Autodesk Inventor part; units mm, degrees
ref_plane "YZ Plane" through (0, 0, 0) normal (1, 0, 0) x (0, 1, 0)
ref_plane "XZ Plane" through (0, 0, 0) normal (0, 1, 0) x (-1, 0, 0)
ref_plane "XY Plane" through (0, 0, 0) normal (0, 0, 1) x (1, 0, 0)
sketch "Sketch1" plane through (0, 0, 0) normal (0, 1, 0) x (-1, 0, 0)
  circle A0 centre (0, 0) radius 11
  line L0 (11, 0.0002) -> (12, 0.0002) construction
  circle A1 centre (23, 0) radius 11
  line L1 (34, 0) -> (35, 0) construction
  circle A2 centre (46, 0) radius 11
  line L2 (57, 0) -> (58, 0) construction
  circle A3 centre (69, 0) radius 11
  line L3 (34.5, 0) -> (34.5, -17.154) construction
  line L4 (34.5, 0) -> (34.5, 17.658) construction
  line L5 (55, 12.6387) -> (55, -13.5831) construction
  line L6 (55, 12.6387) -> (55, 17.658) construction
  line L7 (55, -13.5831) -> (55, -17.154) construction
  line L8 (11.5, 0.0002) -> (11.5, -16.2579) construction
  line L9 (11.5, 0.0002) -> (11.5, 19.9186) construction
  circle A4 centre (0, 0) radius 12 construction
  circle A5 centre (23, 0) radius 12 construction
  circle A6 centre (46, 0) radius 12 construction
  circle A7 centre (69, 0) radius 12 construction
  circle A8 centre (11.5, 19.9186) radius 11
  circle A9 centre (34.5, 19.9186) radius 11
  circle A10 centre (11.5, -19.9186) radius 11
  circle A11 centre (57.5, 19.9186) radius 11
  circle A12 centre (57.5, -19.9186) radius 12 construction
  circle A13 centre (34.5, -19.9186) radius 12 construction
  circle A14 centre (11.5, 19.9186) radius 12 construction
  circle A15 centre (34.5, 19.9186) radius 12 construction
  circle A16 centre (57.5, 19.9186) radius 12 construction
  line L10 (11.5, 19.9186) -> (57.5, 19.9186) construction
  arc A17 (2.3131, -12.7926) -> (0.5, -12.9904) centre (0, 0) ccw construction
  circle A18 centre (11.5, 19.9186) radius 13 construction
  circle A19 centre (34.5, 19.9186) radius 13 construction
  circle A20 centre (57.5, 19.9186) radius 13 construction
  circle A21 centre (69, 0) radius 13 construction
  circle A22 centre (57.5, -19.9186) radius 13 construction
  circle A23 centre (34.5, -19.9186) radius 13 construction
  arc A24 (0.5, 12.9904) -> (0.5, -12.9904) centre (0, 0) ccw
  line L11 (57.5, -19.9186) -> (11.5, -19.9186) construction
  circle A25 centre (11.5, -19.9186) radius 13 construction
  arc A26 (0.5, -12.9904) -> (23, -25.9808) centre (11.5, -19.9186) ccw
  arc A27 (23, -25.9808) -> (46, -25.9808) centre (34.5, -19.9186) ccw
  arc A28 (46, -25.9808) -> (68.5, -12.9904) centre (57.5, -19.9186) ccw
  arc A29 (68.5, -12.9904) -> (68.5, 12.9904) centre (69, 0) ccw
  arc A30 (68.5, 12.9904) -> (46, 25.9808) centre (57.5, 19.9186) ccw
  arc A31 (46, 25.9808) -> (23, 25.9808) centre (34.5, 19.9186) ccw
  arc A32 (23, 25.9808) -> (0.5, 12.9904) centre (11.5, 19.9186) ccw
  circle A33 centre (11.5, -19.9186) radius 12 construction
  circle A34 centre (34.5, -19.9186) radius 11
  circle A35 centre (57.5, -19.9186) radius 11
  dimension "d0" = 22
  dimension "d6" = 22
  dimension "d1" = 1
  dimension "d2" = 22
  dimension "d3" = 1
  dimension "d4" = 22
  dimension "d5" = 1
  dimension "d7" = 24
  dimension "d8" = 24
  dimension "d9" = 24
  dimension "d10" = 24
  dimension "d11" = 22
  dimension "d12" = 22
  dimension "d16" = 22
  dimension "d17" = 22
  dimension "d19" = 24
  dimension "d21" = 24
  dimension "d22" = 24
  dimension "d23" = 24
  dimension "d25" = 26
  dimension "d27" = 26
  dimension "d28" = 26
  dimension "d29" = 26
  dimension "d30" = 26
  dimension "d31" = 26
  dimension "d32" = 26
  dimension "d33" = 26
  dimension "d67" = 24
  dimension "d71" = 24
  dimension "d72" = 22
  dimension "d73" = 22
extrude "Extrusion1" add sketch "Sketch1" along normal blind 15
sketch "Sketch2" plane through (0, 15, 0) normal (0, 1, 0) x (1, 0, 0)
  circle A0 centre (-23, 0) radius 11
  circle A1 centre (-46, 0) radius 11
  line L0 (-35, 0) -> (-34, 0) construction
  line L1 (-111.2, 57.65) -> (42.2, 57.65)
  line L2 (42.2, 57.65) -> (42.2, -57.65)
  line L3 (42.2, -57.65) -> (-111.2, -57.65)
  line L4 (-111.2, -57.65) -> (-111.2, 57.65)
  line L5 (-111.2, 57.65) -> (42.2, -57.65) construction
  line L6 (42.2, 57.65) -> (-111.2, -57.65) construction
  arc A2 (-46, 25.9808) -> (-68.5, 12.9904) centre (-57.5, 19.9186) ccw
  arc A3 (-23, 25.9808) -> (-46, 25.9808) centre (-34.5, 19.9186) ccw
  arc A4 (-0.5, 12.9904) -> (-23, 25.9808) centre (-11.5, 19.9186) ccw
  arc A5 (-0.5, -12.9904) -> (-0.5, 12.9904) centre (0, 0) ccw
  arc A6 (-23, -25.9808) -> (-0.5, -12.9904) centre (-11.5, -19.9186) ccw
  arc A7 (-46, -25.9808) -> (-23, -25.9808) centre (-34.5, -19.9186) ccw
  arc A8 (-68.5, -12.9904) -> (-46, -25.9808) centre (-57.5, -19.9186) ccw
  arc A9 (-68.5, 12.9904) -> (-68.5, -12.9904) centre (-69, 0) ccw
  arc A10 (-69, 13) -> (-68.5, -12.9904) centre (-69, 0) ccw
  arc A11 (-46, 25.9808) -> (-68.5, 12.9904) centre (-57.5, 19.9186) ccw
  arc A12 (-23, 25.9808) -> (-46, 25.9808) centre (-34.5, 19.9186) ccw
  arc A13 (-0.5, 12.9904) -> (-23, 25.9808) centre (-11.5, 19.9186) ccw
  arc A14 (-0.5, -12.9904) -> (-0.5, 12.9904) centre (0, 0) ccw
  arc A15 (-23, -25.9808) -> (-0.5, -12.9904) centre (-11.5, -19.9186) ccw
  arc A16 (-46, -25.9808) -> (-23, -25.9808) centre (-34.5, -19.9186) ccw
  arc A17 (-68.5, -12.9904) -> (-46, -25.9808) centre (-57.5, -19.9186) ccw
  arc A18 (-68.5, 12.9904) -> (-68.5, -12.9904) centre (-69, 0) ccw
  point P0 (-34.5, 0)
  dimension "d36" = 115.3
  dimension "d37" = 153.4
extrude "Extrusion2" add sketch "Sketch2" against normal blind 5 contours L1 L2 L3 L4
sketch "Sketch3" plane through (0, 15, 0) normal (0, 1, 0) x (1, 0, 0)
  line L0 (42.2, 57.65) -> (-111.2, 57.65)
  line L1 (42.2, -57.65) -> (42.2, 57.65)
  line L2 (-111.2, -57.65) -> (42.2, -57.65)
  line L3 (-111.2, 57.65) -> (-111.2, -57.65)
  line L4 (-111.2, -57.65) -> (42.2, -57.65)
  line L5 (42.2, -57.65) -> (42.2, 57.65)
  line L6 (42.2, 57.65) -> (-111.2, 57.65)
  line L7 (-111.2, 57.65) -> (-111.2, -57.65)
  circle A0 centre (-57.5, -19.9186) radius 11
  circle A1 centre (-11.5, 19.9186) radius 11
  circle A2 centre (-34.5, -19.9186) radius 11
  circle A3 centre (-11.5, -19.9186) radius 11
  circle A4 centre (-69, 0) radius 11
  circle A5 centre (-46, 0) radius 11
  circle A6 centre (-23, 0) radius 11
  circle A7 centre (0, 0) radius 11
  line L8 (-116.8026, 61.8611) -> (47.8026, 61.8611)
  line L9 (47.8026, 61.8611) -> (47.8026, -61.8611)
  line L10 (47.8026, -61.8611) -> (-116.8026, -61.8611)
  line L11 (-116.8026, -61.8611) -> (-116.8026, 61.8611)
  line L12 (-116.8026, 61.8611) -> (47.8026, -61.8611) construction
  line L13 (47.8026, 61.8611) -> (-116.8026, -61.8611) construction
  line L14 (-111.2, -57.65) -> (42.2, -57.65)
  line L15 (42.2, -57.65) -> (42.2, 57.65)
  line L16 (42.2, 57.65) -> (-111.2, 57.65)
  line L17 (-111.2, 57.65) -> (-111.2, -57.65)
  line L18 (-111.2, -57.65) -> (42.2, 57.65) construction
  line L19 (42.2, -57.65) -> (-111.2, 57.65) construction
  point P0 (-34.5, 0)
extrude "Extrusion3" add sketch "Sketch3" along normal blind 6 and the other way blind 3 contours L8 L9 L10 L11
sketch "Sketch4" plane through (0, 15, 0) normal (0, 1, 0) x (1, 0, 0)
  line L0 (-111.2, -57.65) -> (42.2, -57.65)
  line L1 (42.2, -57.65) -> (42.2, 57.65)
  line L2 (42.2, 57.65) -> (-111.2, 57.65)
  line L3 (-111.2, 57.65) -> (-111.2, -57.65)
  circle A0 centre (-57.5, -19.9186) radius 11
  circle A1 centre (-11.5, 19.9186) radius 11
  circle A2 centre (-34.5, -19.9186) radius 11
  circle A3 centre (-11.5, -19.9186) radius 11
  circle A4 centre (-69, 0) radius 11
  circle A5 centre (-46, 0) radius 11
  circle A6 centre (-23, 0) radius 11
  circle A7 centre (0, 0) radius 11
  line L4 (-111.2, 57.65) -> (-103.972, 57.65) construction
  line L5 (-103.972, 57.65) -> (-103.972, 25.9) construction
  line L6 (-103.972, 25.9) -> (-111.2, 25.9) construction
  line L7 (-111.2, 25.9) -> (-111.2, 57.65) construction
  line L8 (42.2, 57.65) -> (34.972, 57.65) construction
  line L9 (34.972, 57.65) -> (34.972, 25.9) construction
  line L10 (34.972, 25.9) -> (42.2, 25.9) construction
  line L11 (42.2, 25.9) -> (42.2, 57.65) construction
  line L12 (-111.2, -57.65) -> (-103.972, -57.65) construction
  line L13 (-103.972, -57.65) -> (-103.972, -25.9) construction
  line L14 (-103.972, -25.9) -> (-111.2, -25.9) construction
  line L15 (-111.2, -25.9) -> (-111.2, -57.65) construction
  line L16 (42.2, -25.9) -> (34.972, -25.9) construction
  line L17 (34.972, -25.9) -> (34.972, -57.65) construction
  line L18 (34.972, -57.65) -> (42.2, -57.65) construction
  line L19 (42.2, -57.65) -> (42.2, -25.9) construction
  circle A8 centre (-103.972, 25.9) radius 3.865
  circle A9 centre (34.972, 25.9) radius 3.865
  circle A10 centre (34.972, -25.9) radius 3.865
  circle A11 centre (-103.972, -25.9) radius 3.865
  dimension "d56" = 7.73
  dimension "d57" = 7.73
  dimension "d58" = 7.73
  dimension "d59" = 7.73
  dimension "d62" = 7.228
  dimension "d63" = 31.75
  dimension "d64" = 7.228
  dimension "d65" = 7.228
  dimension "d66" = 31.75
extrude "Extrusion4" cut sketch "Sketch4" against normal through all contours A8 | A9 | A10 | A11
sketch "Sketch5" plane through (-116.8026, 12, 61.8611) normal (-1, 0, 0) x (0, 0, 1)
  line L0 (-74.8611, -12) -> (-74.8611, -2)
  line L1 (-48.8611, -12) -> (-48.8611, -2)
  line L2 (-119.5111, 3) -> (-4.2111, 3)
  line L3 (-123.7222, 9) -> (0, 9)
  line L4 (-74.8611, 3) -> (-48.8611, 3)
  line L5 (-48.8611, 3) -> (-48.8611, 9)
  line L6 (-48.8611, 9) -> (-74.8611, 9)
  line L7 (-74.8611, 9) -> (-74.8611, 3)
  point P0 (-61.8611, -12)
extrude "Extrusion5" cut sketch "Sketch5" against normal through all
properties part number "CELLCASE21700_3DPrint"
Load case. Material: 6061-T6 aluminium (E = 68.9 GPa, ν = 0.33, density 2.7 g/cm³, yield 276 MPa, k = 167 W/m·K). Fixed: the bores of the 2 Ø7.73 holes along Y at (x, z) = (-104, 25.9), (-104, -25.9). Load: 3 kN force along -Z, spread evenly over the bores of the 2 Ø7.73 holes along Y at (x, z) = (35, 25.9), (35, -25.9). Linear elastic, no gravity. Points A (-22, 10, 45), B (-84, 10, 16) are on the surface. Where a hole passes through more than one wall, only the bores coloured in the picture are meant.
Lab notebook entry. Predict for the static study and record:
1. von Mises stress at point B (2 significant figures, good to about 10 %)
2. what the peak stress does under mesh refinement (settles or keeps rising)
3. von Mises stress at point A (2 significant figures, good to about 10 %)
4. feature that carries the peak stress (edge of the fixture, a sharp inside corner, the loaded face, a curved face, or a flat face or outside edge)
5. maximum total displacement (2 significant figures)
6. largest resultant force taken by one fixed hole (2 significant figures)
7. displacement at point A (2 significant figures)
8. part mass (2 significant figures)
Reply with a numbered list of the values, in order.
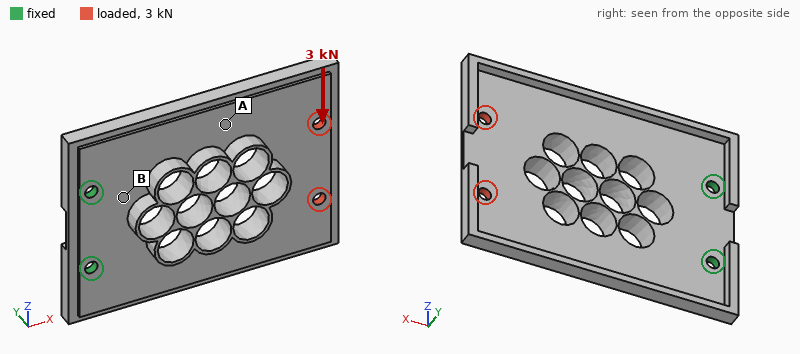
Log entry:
1. 34 MPa
2. keeps rising
3. 14 MPa
4. edge of the fixture
5. 0.51 mm
6. 7.1 kN
7. 0.25 mm
8. 270 g
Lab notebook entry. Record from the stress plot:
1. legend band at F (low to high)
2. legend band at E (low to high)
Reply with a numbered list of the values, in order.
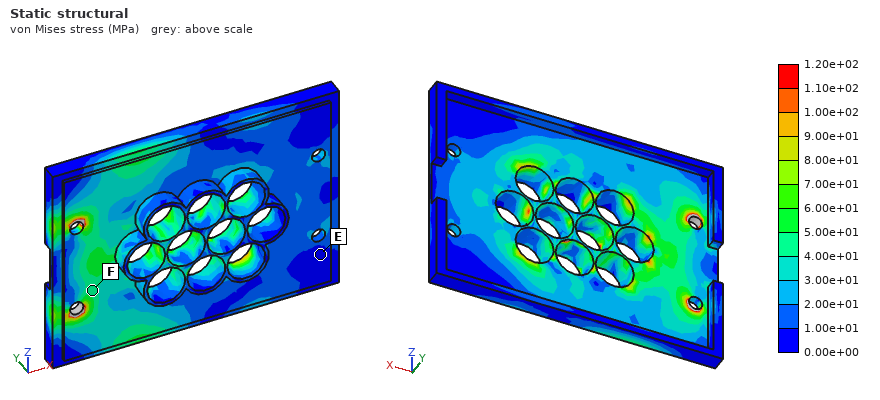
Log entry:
1. 4.00e+01 to 5.00e+01 MPa
2. 0.00e+00 to 1.00e+01 MPa
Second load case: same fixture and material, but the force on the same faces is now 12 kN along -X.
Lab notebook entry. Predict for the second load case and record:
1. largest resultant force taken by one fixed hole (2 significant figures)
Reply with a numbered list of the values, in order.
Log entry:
1. 6.3 kN
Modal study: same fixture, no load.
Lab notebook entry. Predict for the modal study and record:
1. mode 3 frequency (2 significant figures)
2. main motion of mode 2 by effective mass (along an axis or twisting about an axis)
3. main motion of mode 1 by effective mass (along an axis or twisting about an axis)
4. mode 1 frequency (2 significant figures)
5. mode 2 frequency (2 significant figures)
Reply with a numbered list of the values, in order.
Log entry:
1. 1300 Hz
2. twisting about X
3. along Y
4. 210 Hz
5. 450 Hz
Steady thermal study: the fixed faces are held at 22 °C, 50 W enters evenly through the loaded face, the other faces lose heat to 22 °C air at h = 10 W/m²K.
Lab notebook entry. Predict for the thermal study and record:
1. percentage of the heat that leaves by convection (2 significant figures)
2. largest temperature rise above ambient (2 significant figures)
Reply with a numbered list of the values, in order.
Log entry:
1. 36 %
2. 73 K
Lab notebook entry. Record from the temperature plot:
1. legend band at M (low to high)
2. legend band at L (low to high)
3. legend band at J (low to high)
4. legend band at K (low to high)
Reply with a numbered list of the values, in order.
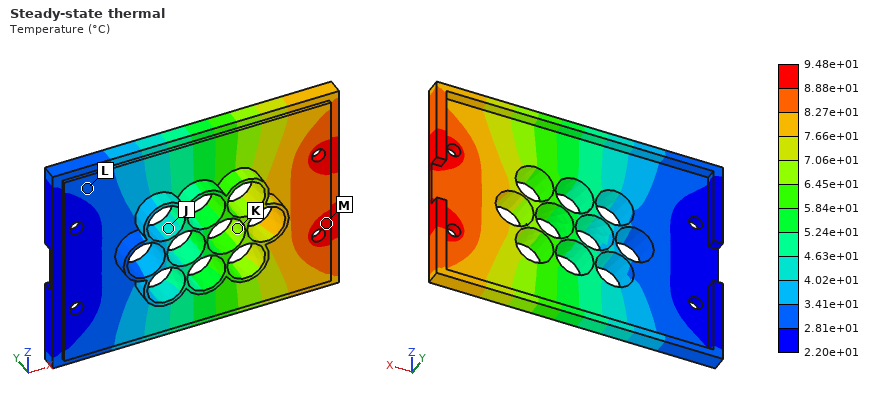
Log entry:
1. 8.88e+01 to 9.48e+01 °C
2. 2.81e+01 to 3.41e+01 °C
3. 4.02e+01 to 4.63e+01 °C
4. 6.45e+01 to 7.06e+01 °C
